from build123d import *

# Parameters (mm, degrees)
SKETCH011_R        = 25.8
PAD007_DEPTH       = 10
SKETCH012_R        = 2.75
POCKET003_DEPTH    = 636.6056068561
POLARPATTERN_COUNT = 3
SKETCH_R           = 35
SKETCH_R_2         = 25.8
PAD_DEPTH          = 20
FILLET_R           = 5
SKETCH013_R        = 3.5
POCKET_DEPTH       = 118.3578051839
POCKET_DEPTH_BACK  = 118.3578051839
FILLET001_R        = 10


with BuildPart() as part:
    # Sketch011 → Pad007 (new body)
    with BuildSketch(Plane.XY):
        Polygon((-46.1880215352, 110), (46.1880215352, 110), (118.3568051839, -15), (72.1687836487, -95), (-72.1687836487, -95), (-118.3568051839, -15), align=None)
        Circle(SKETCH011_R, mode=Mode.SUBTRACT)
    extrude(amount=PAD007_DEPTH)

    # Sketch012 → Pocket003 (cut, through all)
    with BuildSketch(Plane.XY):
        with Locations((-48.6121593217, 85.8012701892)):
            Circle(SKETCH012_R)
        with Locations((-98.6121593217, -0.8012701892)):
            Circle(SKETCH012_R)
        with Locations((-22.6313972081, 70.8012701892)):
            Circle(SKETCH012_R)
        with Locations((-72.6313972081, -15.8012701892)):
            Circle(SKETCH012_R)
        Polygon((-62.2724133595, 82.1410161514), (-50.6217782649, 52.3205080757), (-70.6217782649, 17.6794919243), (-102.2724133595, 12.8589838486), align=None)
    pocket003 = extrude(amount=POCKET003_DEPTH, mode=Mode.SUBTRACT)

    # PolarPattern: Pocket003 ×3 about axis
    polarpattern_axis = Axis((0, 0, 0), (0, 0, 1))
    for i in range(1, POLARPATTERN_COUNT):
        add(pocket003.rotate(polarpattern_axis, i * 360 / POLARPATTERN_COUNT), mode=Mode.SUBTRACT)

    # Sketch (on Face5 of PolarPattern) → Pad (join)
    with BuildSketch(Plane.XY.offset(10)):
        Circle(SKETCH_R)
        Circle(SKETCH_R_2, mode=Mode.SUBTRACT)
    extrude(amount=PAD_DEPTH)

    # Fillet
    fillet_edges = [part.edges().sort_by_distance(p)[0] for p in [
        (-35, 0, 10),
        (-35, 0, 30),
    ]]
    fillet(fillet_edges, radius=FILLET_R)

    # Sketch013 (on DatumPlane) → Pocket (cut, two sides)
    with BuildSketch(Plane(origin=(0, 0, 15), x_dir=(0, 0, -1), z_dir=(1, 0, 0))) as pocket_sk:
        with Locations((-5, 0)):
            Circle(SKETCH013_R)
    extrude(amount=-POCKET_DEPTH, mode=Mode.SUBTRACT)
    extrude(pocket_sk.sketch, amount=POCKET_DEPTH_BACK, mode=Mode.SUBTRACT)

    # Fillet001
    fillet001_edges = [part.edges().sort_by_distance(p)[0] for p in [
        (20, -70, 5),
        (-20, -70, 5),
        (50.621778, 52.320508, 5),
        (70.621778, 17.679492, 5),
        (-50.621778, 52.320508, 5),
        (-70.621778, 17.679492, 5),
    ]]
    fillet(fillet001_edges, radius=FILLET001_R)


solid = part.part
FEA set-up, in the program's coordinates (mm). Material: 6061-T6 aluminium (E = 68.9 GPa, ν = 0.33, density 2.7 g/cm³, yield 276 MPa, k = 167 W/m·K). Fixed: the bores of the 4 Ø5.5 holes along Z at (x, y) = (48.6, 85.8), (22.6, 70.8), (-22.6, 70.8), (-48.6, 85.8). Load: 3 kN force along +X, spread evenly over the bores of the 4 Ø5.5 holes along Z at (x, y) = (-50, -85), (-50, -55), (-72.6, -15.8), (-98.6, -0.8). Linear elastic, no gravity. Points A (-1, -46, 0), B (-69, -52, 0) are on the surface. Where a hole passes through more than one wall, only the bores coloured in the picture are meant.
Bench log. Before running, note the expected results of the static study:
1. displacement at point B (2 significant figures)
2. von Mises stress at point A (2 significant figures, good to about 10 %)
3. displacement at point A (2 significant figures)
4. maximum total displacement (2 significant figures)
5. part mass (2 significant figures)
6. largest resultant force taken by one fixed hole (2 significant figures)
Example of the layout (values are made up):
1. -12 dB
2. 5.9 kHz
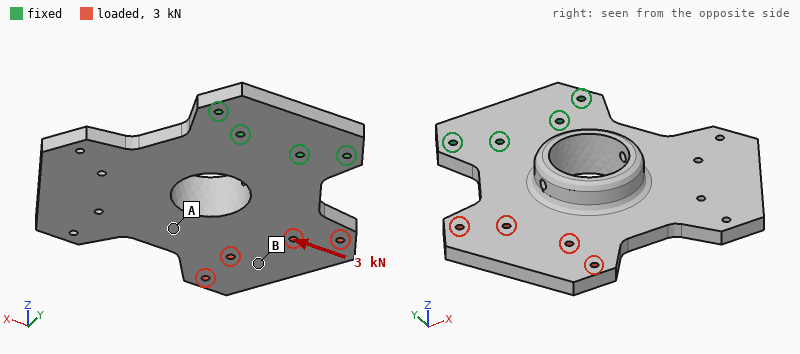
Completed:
1. 68 µm
2. 8.7 MPa
3. 52 µm
4. 87 µm
5. 870 g
6. 2.6 kN
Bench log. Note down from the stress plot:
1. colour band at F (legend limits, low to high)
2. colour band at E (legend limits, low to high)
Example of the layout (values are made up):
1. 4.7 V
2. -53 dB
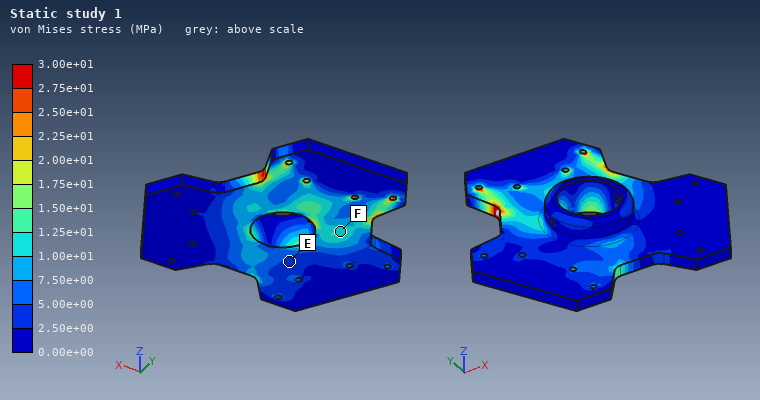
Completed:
1. 1.00e+01 to 1.25e+01 MPa
2. 2.50e+00 to 5.00e+00 MPa
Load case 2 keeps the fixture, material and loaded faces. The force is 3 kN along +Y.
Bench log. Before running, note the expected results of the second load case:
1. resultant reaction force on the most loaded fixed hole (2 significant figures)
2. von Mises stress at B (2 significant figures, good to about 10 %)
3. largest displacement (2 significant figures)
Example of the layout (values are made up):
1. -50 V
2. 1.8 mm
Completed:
1. 2.2 kN
2. 2.2 MPa
3. 48 µm
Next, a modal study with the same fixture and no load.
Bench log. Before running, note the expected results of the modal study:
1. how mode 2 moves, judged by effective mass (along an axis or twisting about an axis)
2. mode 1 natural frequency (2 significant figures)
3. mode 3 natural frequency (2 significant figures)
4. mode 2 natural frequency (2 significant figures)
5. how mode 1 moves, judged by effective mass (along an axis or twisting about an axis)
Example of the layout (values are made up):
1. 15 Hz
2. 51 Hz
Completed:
1. twisting about Y
2. 270 Hz
3. 1300 Hz
4. 510 Hz
5. along Z
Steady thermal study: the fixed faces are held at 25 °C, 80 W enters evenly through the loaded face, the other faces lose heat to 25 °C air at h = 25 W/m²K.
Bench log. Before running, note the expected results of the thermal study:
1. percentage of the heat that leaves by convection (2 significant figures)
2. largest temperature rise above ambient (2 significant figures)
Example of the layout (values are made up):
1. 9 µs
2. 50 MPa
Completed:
1. 42 %
2. 46 K
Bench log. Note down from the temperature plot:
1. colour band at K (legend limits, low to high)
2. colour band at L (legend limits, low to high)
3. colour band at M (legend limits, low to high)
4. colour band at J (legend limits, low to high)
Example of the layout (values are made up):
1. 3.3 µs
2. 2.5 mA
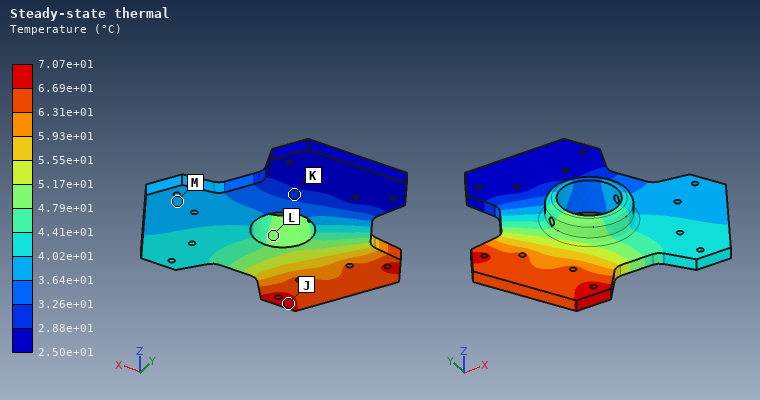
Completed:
1. 2.88e+01 to 3.26e+01 °C
2. 4.79e+01 to 5.17e+01 °C
3. 3.64e+01 to 4.02e+01 °C
4. 6.69e+01 to 7.07e+01 °C
